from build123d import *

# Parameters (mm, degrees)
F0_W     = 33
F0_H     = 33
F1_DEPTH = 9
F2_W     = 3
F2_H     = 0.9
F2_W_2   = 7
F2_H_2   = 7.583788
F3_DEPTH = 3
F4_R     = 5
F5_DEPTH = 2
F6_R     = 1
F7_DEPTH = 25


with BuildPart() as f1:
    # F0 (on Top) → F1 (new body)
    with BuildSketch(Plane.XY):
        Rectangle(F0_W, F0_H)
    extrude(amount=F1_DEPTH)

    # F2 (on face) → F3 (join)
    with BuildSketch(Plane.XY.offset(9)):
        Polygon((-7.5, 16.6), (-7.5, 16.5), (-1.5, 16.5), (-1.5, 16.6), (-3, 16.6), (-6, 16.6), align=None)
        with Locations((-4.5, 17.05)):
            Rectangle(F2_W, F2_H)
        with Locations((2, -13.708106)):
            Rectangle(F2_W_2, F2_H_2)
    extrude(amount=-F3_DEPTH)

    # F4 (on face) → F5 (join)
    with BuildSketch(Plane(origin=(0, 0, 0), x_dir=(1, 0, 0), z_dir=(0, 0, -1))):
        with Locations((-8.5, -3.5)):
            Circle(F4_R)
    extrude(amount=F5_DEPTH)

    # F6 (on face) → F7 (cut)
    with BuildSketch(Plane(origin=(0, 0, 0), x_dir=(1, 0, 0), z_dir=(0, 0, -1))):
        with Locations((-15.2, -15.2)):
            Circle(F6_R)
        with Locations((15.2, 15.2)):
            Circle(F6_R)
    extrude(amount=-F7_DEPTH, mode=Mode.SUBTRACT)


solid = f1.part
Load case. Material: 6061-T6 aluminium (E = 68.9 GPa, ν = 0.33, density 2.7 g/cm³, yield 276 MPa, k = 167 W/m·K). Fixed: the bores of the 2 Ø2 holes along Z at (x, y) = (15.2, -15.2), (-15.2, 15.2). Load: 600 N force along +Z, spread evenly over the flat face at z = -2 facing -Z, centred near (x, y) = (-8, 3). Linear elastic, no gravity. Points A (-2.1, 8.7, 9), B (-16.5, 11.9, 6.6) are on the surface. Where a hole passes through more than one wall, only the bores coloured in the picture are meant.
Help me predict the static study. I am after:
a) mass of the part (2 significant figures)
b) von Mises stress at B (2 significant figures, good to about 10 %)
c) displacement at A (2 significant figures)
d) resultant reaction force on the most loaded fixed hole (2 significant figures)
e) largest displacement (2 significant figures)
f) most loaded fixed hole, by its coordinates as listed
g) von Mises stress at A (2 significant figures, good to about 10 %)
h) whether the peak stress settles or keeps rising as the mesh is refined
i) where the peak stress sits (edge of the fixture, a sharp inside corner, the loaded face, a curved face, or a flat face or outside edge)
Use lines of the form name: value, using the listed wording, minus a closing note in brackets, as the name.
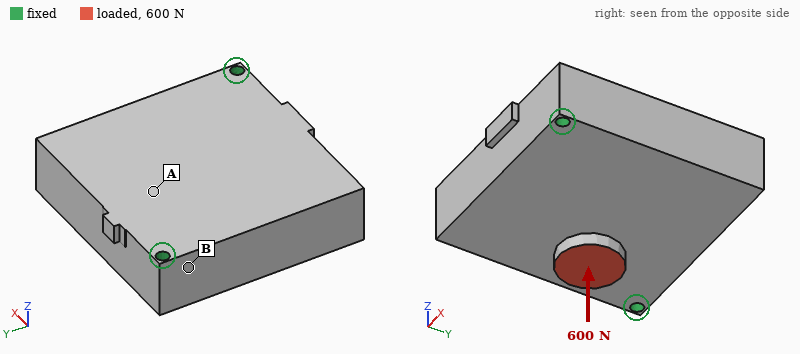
mass of the part: 27 g
von Mises stress at B: 24 MPa
displacement at A: 3.0 µm
resultant reaction force on the most loaded fixed hole: 440 N
largest displacement: 14 µm
most loaded fixed hole, by its coordinates as listed: (-15.2, 15.2)
von Mises stress at A: 7.1 MPa
whether the peak stress settles or keeps rising as the mesh is refined: keeps rising
where the peak stress sits: edge of the fixture
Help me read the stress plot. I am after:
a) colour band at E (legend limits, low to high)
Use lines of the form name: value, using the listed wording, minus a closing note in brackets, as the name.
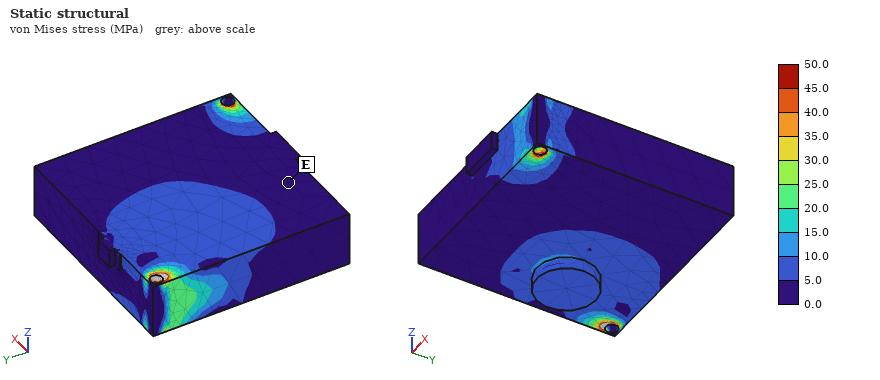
colour band at E: 0.0 to 5.0 MPa
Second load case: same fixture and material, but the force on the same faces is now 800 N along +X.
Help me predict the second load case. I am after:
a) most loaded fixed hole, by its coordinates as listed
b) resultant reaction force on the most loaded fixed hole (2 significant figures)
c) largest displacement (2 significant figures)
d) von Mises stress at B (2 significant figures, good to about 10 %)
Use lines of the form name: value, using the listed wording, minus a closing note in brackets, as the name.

most loaded fixed hole, by its coordinates as listed: (-15.2, 15.2)
resultant reaction force on the most loaded fixed hole: 490 N
largest displacement: 16 µm
von Mises stress at B: 25 MPa
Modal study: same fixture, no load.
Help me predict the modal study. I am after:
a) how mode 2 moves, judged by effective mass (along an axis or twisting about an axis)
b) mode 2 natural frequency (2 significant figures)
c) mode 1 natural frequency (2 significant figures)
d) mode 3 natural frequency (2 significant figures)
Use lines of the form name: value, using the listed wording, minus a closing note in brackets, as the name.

how mode 2 moves, judged by effective mass: along Z
mode 2 natural frequency: 11 kHz
mode 1 natural frequency: 7400 Hz
mode 3 natural frequency: 18 kHz
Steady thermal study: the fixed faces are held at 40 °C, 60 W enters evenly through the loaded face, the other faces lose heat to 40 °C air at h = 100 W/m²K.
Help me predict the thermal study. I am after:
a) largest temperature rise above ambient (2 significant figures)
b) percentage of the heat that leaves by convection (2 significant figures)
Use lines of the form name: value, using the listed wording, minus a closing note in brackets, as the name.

largest temperature rise above ambient: 44 K
percentage of the heat that leaves by convection: 9.9 %
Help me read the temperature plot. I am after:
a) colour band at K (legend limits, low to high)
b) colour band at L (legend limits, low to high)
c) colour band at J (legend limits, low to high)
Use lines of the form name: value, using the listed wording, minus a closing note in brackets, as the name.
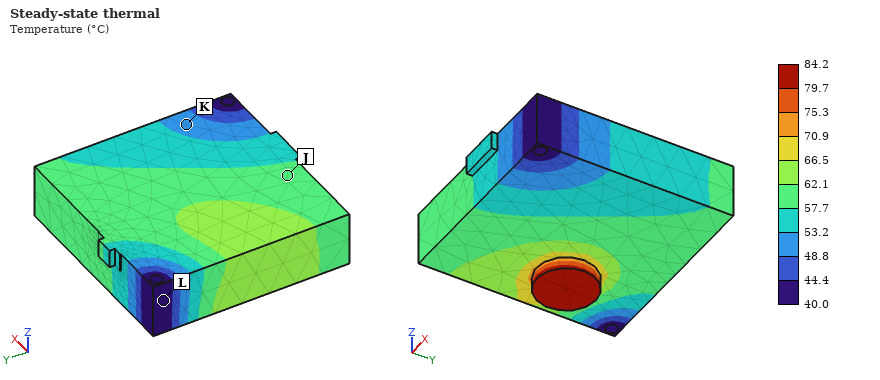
colour band at K: 48.8 to 53.2 °C
colour band at L: 40.0 to 44.4 °C
colour band at J: 57.7 to 62.1 °C
